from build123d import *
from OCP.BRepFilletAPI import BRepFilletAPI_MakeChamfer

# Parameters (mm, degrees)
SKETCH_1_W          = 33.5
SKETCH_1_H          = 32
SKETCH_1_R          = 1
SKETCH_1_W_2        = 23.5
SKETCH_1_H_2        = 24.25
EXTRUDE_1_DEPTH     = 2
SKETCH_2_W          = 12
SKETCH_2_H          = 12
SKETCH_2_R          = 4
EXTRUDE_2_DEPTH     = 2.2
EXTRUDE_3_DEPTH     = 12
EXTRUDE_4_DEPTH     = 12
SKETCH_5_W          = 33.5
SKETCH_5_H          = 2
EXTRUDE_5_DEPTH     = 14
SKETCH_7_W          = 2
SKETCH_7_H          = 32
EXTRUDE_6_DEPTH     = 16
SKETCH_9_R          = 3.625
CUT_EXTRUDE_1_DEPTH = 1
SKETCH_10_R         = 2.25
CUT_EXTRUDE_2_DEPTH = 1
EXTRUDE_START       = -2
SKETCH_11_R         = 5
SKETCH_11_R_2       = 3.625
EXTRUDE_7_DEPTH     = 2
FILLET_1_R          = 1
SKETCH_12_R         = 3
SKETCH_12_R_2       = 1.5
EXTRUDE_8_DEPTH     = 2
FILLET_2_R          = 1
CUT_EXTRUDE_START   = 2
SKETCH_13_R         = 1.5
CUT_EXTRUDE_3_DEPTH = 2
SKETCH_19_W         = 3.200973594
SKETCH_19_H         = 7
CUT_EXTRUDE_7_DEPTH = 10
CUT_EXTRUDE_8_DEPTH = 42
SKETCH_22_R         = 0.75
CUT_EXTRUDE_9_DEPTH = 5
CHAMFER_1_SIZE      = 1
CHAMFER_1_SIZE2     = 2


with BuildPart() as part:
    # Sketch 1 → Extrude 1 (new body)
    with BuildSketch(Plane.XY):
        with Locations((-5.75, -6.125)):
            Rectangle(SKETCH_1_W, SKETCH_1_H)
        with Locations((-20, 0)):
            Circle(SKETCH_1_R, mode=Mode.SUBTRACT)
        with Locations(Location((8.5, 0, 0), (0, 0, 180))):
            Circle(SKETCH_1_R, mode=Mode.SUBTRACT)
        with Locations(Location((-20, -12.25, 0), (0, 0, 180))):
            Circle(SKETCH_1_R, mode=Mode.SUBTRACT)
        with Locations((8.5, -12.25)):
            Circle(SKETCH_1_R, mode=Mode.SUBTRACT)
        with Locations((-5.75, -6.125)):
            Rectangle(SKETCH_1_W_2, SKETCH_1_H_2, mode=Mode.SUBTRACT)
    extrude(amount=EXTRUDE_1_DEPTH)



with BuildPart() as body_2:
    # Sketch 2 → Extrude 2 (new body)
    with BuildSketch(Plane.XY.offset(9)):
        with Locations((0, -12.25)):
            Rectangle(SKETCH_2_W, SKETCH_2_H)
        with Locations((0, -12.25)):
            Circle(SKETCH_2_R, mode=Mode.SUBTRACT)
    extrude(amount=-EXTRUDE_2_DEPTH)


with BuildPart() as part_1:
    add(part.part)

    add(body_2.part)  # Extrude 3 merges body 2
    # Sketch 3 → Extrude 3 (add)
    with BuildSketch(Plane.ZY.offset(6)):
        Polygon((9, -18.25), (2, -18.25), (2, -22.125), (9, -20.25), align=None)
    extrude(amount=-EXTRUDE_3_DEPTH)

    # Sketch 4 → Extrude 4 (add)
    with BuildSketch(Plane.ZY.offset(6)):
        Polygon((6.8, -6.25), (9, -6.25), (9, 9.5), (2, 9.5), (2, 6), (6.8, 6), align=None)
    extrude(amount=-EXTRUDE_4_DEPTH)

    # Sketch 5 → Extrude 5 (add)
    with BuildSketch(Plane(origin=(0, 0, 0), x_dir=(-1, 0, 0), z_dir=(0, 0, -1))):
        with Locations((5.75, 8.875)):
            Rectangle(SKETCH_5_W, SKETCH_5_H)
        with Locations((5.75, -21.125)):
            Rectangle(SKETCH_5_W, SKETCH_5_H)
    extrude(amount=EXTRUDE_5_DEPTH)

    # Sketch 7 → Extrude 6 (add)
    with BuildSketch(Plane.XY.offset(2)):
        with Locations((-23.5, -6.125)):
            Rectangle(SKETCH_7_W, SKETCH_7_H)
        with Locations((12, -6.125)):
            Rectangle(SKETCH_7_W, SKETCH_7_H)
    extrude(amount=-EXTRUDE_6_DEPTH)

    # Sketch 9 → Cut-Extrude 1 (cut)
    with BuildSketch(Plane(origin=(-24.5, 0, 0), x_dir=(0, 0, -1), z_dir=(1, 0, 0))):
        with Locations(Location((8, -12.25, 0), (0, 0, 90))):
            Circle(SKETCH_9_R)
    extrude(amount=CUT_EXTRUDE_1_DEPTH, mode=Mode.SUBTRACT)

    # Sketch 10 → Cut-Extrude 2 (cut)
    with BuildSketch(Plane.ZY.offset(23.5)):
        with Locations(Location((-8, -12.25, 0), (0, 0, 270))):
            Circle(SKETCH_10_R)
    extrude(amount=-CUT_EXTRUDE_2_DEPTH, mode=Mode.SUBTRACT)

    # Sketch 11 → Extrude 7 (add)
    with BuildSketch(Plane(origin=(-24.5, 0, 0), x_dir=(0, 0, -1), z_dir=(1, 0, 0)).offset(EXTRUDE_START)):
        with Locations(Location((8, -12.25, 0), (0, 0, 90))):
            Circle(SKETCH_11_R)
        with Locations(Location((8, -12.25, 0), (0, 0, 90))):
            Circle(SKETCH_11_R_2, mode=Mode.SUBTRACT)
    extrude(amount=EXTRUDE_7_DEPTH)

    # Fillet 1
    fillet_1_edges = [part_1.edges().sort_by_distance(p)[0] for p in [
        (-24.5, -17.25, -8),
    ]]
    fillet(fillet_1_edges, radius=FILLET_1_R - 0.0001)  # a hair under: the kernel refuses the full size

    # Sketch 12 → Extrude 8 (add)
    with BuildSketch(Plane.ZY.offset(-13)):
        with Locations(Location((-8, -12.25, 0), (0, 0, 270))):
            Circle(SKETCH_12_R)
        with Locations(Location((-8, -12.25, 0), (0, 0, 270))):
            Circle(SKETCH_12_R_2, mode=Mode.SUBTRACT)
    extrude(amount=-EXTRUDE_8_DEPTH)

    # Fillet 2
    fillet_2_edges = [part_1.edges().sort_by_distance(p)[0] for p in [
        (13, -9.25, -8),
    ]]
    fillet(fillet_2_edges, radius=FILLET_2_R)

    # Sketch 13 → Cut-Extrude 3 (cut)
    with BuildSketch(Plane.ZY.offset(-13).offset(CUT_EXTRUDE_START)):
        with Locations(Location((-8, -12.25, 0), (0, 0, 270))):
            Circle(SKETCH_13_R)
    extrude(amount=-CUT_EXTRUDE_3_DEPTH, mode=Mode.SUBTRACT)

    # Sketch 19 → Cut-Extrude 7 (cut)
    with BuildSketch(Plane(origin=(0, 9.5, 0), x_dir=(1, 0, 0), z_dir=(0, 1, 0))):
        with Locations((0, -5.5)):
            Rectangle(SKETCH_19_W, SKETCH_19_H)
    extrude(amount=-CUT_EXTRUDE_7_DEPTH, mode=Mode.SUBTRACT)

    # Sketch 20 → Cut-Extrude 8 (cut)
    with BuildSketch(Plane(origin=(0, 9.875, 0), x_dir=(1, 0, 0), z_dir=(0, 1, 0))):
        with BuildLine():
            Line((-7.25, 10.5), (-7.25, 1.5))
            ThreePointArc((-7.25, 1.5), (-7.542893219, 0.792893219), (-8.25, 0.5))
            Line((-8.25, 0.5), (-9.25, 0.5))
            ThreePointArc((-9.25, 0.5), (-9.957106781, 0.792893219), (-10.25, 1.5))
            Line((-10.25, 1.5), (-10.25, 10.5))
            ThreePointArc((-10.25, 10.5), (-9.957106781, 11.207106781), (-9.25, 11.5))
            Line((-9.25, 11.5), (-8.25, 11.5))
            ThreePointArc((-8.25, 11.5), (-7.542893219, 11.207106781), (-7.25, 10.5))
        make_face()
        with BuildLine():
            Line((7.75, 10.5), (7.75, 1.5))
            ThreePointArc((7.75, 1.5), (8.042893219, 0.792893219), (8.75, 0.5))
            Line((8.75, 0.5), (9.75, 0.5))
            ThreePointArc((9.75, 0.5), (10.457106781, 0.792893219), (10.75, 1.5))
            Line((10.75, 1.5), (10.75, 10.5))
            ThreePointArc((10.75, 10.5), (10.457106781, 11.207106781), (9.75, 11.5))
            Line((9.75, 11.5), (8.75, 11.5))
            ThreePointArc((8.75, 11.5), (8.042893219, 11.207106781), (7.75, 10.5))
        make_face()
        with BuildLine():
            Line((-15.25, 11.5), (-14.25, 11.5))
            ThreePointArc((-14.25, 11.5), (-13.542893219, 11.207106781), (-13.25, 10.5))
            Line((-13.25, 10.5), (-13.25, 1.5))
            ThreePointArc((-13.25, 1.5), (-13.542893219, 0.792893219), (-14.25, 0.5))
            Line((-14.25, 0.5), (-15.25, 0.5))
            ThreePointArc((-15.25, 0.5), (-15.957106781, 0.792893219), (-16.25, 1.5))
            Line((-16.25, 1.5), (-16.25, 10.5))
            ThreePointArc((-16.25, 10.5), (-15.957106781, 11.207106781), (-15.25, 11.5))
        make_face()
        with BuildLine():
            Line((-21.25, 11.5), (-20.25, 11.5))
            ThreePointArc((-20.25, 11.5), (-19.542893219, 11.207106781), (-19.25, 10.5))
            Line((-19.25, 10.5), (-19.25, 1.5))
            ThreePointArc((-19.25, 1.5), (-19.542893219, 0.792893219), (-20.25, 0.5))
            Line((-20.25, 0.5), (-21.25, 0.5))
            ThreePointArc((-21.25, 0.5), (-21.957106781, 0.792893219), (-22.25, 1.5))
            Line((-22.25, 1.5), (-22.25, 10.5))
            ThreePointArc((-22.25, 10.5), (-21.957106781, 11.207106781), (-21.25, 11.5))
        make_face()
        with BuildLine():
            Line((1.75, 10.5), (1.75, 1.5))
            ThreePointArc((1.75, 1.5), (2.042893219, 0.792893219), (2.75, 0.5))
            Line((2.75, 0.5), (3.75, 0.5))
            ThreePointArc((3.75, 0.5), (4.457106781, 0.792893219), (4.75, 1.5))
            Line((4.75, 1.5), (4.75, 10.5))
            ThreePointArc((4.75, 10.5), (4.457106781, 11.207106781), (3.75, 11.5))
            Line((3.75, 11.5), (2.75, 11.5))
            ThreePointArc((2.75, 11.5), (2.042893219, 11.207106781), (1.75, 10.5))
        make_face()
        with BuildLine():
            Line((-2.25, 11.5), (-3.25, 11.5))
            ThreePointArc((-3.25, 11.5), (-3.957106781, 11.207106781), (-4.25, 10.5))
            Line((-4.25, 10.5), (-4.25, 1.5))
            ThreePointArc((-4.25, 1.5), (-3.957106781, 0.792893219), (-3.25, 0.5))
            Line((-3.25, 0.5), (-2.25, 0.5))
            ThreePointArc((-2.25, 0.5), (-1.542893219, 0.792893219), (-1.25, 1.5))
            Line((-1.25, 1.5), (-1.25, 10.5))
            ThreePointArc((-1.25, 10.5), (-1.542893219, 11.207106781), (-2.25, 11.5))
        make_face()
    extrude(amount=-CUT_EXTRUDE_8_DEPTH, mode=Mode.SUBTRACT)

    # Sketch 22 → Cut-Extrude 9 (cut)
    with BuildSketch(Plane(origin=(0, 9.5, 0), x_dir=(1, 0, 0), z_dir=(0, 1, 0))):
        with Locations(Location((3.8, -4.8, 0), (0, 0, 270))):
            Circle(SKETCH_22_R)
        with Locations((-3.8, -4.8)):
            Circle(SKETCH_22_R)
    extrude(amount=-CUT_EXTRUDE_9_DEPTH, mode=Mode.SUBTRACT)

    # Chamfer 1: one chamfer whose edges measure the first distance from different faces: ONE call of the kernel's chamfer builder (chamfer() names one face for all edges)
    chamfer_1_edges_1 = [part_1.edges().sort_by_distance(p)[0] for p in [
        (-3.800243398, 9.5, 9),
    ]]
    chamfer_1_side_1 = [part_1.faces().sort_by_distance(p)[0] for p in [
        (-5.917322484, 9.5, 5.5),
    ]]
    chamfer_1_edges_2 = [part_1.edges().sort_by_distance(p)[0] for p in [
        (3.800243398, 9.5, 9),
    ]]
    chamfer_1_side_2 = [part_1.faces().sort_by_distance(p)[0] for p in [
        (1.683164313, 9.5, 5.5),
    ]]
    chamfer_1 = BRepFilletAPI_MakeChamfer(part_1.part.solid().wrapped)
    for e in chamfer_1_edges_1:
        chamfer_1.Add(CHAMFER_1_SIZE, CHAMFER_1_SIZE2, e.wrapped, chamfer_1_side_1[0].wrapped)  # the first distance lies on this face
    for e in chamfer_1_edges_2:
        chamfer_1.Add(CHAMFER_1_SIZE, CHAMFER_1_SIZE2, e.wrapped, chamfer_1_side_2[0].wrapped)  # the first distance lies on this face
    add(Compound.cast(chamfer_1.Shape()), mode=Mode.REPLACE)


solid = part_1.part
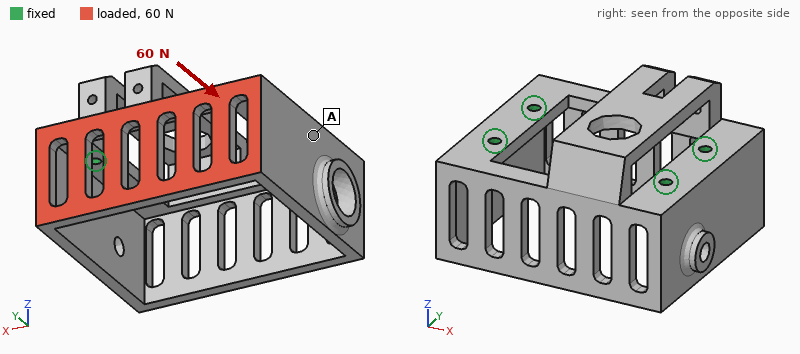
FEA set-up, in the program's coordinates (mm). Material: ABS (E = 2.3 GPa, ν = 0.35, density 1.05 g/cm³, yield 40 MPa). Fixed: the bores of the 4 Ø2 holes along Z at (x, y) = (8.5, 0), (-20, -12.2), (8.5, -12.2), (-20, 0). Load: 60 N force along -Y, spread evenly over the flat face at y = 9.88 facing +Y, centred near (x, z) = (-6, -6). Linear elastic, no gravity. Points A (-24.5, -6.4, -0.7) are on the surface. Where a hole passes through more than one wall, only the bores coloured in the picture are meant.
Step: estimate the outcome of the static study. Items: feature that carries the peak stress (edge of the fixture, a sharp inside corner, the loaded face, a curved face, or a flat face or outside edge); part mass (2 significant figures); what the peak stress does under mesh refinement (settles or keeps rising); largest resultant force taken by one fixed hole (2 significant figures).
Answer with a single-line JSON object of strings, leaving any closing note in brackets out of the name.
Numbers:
{"feature that carries the peak stress": "a sharp inside corner", "part mass": "5.4 g", "what the peak stress does under mesh refinement": "keeps rising", "largest resultant force taken by one fixed hole": "34 N"}
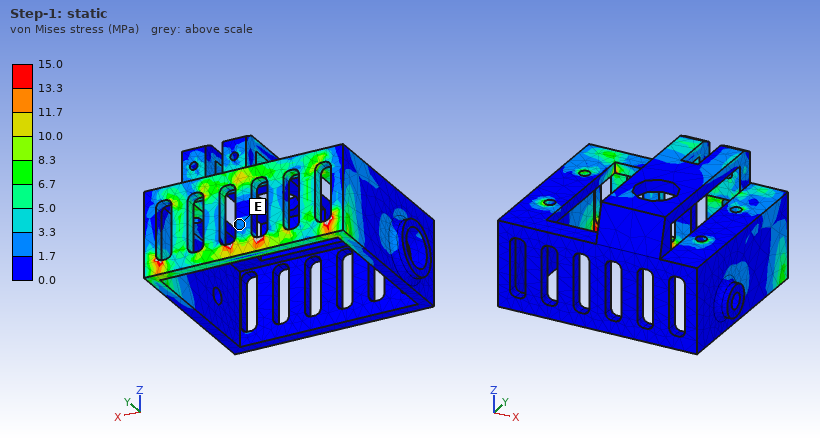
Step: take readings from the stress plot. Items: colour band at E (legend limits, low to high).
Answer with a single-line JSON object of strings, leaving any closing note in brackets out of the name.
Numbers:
{"colour band at E": "1.7 to 3.3 MPa"}
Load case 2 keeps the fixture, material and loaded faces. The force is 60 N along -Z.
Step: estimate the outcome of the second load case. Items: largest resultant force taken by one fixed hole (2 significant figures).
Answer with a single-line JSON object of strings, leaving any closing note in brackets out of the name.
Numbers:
{"largest resultant force taken by one fixed hole": "48 N"}
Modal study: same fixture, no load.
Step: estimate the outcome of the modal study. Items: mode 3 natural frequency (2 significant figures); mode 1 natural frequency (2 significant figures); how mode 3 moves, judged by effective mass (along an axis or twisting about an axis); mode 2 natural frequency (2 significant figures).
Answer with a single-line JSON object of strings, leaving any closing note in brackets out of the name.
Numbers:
{"mode 3 natural frequency": "2500 Hz", "mode 1 natural frequency": "2000 Hz", "how mode 3 moves, judged by effective mass": "along X", "mode 2 natural frequency": "2300 Hz"}
